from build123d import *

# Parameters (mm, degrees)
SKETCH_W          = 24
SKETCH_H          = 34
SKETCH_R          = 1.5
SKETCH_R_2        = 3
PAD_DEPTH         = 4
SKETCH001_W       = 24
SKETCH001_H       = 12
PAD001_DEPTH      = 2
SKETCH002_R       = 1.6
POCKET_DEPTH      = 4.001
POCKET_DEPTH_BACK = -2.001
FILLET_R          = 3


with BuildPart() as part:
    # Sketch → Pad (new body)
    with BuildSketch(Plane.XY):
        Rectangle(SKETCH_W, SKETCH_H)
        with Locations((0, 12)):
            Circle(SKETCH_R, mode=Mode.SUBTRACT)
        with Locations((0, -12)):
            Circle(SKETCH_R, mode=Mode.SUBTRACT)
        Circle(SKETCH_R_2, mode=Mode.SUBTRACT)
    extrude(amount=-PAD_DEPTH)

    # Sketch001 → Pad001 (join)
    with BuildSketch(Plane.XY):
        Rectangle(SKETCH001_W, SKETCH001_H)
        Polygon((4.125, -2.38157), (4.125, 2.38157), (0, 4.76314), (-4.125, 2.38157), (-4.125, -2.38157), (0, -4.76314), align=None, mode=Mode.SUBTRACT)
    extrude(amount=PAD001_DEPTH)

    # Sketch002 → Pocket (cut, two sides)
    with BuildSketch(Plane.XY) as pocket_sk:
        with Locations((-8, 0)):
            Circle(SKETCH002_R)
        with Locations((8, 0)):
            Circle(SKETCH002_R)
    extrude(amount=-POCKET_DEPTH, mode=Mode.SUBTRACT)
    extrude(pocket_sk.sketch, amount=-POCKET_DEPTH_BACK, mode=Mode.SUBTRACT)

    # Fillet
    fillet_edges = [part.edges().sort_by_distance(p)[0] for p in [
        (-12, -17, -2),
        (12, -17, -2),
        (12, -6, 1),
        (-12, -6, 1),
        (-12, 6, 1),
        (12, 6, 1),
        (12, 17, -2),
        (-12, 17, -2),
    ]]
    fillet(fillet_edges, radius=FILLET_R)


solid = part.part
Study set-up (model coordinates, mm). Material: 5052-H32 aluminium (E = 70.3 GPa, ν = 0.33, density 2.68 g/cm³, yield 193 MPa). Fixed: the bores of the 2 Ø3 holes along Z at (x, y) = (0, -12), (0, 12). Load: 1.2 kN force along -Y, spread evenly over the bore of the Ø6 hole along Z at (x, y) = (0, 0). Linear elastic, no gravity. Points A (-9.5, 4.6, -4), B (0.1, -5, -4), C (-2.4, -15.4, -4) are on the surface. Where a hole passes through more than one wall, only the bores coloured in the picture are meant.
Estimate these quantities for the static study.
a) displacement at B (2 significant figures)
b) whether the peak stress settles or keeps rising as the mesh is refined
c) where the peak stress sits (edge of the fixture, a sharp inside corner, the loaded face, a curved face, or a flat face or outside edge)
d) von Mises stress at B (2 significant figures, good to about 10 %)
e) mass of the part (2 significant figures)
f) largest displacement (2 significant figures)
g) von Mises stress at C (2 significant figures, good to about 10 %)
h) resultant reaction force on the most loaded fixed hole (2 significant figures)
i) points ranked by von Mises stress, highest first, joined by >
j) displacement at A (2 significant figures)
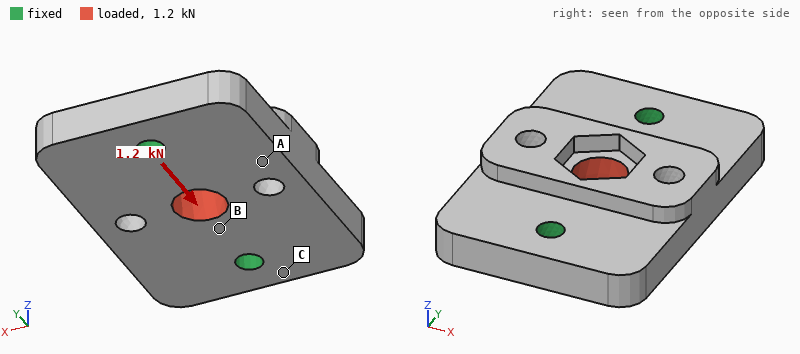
1.6 µm
keeps rising
edge of the fixture
19 MPa
9.1 g
2.5 µm
5.6 MPa
600 N
B > C > A
1.4 µm
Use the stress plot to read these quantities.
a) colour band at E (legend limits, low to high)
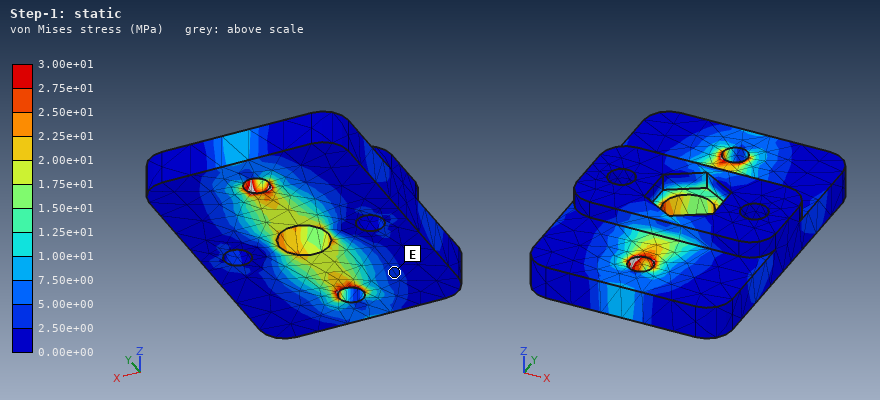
2.50e+00 to 5.00e+00 MPa
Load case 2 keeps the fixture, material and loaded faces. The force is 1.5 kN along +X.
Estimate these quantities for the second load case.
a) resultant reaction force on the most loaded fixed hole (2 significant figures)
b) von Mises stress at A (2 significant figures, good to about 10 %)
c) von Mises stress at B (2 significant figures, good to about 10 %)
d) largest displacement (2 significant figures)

750 N
13 MPa
14 MPa
5.7 µm
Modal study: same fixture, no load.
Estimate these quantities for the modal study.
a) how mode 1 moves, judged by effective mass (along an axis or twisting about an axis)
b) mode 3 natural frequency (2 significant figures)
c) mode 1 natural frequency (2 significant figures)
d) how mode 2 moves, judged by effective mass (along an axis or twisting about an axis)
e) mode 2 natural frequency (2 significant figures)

twisting about Y
28 kHz
15 kHz
along Z
20 kHz
